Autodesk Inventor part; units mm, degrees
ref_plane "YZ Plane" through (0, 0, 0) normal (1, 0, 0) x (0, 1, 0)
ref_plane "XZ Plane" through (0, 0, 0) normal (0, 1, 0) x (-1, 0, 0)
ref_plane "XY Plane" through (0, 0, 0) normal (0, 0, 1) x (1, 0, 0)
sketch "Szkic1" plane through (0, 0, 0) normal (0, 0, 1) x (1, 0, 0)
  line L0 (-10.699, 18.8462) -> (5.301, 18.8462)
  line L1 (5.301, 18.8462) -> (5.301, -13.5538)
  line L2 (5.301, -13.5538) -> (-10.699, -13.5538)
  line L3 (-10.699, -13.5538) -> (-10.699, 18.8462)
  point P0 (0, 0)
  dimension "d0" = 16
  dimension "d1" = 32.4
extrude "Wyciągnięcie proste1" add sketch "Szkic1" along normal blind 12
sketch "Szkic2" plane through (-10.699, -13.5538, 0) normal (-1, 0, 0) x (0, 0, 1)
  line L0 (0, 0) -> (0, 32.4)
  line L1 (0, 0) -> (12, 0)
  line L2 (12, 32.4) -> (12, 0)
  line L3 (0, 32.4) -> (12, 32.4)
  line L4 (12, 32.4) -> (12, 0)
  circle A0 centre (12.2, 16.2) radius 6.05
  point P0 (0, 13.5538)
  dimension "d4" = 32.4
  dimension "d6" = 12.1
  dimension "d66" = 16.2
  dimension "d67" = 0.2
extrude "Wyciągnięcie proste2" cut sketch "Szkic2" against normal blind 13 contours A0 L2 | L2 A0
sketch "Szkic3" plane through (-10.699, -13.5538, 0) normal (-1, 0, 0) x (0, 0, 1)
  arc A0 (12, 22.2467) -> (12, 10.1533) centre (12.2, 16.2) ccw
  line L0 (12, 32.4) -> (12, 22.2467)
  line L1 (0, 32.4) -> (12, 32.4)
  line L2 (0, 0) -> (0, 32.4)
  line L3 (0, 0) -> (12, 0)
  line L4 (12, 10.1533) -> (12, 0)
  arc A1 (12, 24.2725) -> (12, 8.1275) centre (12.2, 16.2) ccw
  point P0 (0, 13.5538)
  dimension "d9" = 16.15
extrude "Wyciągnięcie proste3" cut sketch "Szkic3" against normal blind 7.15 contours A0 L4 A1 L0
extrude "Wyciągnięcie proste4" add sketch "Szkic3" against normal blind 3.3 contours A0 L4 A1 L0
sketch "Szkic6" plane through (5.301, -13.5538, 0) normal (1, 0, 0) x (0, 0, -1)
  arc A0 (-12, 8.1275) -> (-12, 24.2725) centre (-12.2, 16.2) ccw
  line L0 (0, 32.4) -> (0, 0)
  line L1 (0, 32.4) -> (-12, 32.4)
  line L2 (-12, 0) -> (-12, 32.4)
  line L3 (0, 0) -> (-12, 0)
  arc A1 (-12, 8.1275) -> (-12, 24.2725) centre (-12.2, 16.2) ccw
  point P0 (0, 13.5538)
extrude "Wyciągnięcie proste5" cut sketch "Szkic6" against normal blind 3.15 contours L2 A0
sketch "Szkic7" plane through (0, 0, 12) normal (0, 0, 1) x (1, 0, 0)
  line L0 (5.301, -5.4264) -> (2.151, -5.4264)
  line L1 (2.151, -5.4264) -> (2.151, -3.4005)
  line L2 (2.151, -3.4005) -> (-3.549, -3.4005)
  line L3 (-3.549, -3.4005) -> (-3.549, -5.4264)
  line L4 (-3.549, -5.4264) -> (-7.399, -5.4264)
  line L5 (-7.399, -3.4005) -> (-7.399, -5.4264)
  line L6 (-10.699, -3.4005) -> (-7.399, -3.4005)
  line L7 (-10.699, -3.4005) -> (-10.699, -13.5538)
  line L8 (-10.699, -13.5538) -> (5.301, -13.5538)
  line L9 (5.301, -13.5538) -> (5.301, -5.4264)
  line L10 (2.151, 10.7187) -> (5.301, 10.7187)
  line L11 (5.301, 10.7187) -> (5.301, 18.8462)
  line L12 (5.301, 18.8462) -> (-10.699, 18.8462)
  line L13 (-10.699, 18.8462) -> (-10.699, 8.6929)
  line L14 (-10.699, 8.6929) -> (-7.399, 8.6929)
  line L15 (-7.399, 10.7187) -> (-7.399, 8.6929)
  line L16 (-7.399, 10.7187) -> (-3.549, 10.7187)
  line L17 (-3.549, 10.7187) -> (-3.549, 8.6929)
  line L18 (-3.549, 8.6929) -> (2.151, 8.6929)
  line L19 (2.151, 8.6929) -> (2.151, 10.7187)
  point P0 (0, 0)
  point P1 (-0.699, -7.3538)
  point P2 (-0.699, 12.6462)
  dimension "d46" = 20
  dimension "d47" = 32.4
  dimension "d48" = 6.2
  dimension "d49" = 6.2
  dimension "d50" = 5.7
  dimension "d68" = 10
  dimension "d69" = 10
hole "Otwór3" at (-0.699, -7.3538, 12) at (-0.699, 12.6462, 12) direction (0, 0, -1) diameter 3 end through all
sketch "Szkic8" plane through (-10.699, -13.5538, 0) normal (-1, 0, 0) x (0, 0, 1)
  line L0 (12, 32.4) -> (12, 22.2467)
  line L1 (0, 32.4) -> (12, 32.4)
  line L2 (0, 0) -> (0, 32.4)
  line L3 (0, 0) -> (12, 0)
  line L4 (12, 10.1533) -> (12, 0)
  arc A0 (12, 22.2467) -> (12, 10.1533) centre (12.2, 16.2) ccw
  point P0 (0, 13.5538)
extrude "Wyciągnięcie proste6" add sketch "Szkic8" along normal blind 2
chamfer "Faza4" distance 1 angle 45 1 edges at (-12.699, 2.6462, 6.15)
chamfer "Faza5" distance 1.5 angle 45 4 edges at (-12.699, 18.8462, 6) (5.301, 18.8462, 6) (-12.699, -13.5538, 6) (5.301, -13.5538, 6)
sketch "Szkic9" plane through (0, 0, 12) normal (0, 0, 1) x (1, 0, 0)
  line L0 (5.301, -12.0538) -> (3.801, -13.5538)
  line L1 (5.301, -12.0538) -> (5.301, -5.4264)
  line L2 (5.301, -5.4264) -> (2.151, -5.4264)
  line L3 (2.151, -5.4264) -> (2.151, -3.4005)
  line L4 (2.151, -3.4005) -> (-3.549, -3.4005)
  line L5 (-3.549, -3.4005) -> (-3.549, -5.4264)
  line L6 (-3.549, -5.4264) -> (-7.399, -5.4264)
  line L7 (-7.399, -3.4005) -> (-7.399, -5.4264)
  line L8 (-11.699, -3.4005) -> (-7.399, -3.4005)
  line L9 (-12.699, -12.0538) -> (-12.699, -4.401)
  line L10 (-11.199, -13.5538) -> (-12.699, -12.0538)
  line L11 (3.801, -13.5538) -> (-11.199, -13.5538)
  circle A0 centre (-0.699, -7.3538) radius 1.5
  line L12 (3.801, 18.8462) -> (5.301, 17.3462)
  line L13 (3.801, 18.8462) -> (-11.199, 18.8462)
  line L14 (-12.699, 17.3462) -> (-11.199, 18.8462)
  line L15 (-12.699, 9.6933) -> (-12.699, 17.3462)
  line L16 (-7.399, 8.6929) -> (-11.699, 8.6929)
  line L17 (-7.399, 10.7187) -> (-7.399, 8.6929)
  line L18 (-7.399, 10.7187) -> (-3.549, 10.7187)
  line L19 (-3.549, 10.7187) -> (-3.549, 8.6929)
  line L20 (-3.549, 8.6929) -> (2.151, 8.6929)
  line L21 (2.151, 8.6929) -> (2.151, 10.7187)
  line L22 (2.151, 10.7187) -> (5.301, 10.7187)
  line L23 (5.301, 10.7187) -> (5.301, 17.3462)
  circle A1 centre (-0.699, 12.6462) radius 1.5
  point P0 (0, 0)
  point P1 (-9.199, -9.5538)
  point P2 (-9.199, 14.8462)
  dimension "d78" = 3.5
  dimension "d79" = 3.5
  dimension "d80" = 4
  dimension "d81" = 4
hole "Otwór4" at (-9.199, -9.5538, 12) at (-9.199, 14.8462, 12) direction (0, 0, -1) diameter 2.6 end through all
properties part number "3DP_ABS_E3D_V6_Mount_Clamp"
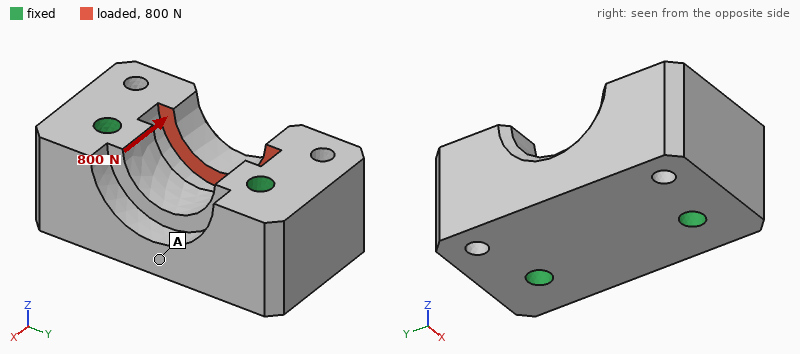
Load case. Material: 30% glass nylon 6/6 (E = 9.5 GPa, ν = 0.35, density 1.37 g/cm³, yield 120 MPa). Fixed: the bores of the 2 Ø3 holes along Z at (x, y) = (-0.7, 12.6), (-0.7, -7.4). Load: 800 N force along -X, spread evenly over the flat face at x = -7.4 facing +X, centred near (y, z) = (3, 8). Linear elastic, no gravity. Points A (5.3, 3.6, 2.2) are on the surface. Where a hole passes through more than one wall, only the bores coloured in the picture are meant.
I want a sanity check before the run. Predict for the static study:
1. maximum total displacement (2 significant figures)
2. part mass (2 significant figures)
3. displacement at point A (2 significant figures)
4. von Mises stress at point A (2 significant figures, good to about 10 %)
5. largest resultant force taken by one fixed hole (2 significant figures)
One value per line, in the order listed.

22 µm
7.3 g
3.9 µm
3.5 MPa
420 N
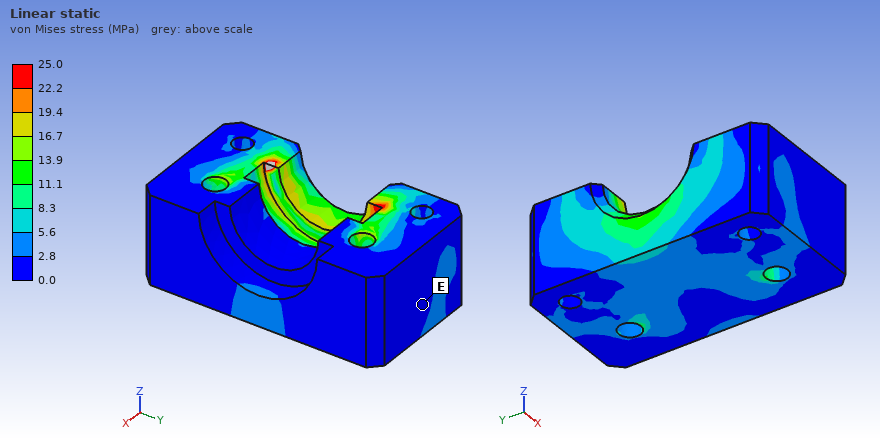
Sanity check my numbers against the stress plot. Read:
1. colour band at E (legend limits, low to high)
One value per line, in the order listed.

0.0 to 2.8 MPa
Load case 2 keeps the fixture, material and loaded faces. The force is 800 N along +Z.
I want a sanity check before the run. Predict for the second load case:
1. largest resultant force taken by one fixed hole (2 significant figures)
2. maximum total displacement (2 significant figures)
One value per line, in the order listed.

410 N
35 µm
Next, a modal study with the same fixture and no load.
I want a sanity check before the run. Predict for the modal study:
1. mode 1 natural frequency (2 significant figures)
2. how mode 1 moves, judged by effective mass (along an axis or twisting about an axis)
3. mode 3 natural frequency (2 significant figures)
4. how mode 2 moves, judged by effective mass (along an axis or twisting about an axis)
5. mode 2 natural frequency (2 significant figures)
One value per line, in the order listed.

19 kHz
along Z
25 kHz
along Y
21 kHz
